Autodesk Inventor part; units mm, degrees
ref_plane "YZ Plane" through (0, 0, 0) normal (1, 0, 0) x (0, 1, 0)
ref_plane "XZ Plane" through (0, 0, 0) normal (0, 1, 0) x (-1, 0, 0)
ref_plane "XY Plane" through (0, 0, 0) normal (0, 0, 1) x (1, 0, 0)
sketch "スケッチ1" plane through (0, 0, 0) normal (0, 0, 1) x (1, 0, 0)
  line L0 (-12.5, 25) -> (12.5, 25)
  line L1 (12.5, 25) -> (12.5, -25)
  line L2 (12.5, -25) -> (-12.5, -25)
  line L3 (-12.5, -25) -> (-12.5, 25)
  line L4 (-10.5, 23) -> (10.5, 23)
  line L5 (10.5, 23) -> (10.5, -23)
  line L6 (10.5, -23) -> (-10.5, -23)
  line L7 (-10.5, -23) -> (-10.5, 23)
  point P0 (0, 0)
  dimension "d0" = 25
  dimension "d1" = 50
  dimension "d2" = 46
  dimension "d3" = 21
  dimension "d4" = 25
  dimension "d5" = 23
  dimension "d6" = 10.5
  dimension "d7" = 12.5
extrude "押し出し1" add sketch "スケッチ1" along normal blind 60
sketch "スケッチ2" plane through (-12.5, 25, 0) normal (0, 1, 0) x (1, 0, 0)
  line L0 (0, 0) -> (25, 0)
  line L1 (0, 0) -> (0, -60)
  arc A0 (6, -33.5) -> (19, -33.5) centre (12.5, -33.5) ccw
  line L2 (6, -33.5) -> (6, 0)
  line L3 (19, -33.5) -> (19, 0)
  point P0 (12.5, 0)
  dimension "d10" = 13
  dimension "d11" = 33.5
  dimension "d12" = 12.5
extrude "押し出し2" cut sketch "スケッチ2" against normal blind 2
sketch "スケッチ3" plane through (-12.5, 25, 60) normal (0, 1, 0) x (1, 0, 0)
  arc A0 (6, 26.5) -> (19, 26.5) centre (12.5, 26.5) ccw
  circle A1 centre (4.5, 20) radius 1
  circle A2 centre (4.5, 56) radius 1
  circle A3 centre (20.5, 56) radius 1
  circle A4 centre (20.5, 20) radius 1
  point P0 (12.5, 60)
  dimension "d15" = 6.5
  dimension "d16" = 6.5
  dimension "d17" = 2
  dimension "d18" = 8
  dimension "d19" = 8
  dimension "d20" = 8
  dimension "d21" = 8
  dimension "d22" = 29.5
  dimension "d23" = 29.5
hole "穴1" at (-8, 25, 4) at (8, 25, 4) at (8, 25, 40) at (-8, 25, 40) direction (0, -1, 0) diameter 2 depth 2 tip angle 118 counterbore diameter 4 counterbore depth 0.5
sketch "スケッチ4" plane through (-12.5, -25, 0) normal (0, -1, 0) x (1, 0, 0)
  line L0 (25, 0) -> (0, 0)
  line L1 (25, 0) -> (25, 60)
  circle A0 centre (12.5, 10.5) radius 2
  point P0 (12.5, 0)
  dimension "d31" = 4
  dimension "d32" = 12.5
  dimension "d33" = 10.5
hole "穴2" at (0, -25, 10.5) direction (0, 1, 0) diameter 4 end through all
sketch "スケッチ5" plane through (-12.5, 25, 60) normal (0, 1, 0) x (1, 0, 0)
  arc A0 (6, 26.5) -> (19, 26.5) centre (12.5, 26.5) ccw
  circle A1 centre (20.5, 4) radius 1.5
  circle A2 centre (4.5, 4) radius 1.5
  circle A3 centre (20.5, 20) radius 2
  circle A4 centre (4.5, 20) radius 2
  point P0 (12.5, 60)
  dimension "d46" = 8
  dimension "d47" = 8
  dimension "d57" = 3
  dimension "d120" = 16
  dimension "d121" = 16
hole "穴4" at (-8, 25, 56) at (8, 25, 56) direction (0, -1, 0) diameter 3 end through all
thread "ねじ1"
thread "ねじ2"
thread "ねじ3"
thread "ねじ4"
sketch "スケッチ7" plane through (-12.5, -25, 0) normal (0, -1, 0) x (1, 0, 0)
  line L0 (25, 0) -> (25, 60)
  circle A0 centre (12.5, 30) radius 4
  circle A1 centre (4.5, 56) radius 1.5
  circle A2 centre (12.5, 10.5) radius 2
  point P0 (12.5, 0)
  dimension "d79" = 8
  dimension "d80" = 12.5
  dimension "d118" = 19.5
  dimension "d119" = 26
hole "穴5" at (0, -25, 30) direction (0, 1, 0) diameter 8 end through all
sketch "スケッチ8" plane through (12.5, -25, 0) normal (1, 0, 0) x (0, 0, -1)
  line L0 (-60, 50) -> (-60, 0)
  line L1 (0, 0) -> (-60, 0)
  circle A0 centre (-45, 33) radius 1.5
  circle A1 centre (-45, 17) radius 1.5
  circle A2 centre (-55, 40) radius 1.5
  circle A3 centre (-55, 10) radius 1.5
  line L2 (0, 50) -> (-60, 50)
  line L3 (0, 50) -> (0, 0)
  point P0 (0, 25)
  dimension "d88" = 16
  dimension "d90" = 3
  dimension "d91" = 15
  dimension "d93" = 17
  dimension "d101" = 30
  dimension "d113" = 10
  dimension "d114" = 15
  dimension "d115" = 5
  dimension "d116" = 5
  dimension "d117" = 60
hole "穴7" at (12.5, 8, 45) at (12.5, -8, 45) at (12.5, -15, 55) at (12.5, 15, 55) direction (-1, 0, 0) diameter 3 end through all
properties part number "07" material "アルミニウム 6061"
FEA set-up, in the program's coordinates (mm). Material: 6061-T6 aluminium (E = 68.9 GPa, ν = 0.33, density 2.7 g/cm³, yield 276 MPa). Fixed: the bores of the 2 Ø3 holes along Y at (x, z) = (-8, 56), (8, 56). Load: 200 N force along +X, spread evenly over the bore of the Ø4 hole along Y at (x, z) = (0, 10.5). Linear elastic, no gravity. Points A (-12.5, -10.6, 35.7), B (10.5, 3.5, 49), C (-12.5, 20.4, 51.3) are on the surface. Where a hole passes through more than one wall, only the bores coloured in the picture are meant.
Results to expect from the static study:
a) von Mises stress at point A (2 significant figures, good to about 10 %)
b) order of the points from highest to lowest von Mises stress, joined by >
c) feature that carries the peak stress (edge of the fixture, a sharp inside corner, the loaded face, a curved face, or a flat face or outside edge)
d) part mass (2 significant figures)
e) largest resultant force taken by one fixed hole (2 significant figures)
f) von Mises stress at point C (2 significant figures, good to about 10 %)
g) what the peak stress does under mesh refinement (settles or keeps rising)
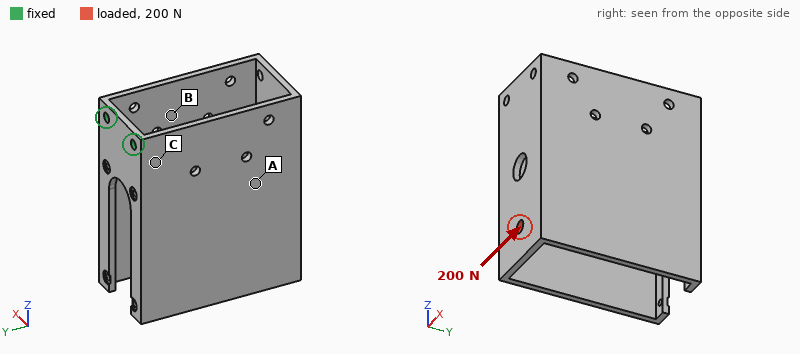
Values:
36 MPa
C > A > B
edge of the fixture
42 g
630 N
78 MPa
keeps rising
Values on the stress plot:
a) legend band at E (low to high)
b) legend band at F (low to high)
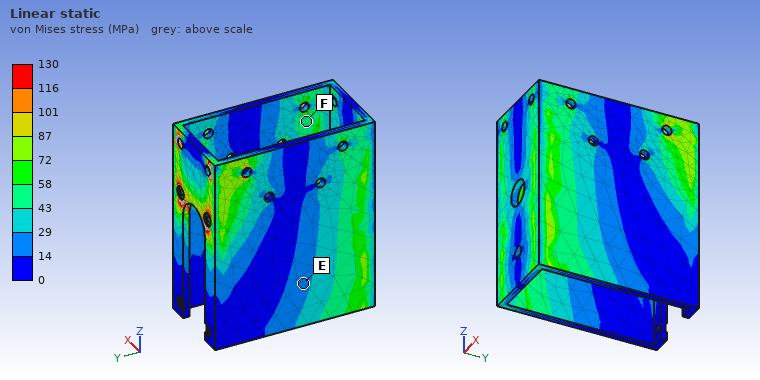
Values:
14 to 29 MPa
43 to 58 MPa
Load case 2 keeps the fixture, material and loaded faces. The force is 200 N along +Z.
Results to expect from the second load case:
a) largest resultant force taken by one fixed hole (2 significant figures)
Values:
100 N
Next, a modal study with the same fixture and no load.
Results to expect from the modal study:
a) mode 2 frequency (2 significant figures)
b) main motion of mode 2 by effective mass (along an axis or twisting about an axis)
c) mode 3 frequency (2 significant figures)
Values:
570 Hz
along X
1100 Hz
